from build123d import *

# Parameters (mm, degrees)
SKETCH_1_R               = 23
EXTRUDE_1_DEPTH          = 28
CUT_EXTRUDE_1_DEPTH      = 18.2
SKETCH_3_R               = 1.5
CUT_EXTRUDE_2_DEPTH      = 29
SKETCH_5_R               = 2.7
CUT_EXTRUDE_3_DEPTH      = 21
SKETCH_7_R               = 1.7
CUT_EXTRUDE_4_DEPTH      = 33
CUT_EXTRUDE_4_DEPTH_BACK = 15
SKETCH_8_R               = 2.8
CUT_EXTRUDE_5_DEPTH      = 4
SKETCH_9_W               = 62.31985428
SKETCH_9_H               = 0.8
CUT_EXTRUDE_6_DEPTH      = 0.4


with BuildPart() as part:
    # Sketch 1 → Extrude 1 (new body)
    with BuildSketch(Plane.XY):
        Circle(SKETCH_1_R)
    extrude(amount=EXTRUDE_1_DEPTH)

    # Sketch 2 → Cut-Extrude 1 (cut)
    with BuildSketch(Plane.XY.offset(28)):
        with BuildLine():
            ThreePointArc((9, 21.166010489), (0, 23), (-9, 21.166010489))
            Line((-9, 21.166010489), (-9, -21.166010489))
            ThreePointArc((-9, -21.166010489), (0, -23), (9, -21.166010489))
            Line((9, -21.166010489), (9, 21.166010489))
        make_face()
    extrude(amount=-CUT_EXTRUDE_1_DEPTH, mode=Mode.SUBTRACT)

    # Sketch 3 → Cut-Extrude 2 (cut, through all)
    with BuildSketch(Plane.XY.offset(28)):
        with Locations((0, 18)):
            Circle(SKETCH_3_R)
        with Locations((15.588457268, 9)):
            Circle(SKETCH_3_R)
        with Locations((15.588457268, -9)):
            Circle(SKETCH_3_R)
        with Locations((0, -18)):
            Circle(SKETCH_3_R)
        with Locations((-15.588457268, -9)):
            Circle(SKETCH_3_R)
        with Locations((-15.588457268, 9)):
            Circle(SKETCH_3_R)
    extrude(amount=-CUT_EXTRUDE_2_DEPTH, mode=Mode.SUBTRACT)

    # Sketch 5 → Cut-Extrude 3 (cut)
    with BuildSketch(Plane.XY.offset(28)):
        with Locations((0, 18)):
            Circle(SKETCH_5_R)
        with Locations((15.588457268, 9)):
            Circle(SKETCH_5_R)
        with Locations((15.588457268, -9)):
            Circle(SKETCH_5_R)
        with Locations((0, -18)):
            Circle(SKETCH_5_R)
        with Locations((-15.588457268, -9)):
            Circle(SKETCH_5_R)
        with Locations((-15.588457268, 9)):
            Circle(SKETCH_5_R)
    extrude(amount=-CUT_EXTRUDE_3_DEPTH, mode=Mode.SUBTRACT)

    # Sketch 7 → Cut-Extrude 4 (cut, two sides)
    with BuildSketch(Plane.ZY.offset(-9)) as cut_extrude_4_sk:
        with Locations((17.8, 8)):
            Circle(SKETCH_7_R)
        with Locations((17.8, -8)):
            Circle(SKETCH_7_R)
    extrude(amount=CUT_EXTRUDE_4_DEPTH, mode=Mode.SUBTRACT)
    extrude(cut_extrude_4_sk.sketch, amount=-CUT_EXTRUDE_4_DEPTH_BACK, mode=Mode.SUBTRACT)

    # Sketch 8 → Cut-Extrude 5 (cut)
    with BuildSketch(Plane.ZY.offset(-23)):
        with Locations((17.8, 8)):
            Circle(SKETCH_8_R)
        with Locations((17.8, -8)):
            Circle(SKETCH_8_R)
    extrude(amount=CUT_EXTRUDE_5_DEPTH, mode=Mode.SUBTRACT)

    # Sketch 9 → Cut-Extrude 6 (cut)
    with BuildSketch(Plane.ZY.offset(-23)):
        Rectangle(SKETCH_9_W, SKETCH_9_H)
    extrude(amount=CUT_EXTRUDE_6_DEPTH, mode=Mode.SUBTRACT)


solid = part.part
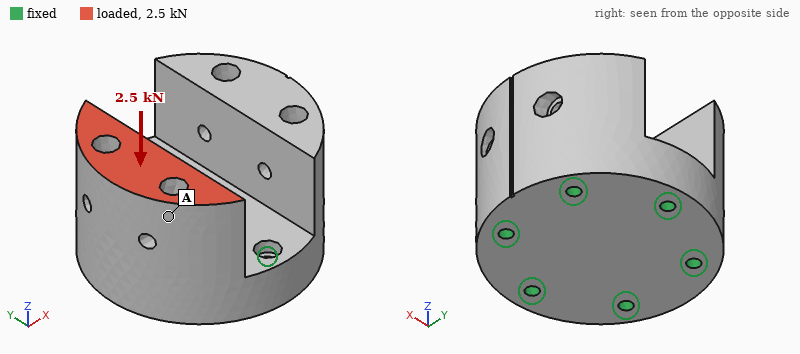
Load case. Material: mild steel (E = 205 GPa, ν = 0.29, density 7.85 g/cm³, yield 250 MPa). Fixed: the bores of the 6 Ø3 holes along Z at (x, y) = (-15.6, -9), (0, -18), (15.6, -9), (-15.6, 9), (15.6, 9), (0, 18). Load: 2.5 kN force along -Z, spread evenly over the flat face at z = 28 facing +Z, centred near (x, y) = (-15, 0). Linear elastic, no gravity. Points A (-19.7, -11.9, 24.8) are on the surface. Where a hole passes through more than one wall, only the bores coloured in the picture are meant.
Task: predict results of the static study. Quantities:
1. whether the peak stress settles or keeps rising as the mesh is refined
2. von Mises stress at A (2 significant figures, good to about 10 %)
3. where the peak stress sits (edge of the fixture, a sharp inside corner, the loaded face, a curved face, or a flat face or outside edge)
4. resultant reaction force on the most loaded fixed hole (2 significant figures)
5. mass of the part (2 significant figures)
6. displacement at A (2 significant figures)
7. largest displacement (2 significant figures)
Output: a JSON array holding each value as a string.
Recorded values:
["keeps rising", "6.8 MPa", "edge of the fixture", "1.1 kN", "230 g", "1.4 µm", "1.6 µm"]
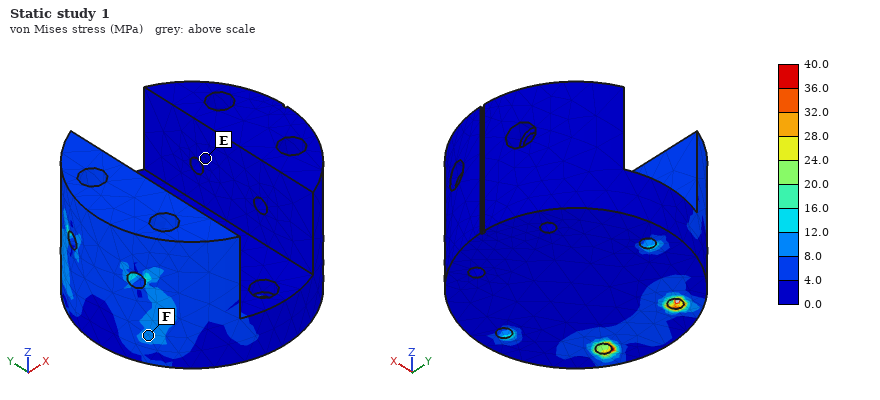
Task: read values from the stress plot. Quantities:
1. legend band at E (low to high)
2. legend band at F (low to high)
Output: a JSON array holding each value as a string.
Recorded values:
["0.0 to 4.0 MPa", "8.0 to 12.0 MPa"]
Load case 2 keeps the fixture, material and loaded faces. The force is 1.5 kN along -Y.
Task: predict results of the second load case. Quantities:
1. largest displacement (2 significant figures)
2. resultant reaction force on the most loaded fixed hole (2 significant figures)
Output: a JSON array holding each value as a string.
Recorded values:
["4.7 µm", "1.1 kN"]
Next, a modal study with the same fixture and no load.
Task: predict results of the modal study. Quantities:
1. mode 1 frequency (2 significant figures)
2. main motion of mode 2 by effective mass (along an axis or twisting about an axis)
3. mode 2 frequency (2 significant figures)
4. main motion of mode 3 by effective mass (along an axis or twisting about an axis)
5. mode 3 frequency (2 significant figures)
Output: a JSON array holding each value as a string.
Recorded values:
["13 kHz", "along X", "14 kHz", "along Y", "19 kHz"]
